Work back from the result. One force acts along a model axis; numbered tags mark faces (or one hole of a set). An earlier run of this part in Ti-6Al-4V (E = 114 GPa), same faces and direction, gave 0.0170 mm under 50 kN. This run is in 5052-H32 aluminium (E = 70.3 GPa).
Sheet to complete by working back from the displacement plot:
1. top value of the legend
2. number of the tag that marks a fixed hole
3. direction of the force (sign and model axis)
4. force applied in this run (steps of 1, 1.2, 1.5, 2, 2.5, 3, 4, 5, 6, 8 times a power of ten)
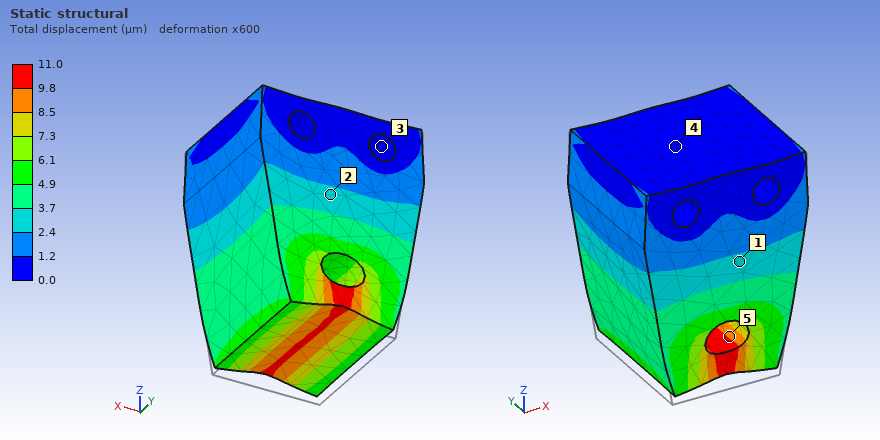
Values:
11.0 µm
3
+Z
20 kN
